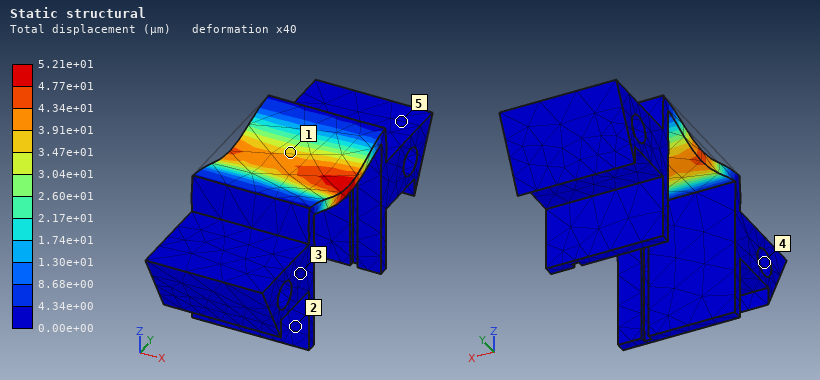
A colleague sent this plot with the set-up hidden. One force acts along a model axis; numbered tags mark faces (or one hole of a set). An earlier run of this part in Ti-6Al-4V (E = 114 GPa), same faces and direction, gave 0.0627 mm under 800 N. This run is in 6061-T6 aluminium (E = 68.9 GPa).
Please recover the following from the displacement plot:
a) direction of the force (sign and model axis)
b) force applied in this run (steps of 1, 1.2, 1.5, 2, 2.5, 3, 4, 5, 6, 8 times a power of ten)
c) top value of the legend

-Z
400 N
5.21e+01 µm
